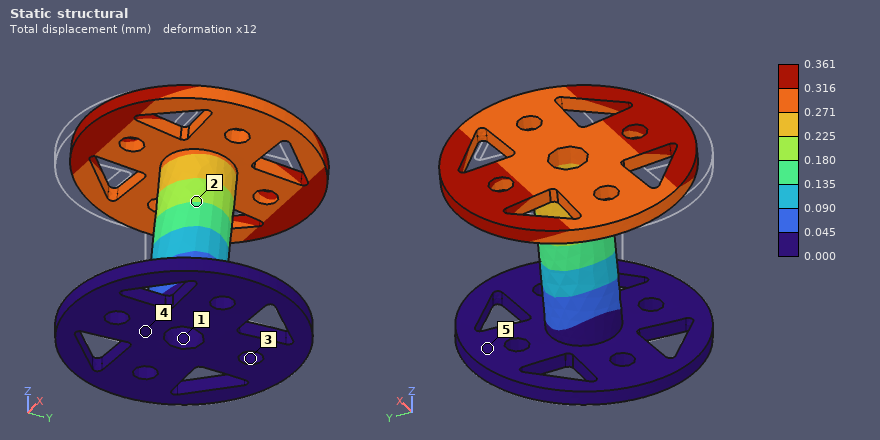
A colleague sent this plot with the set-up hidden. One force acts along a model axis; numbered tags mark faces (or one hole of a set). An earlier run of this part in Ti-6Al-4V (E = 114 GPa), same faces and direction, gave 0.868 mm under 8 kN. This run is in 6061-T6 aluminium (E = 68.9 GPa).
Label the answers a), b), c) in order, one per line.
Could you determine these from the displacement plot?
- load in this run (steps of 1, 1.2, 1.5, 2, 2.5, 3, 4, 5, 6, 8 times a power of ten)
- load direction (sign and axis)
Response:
a) 2 kN
b) +Y
